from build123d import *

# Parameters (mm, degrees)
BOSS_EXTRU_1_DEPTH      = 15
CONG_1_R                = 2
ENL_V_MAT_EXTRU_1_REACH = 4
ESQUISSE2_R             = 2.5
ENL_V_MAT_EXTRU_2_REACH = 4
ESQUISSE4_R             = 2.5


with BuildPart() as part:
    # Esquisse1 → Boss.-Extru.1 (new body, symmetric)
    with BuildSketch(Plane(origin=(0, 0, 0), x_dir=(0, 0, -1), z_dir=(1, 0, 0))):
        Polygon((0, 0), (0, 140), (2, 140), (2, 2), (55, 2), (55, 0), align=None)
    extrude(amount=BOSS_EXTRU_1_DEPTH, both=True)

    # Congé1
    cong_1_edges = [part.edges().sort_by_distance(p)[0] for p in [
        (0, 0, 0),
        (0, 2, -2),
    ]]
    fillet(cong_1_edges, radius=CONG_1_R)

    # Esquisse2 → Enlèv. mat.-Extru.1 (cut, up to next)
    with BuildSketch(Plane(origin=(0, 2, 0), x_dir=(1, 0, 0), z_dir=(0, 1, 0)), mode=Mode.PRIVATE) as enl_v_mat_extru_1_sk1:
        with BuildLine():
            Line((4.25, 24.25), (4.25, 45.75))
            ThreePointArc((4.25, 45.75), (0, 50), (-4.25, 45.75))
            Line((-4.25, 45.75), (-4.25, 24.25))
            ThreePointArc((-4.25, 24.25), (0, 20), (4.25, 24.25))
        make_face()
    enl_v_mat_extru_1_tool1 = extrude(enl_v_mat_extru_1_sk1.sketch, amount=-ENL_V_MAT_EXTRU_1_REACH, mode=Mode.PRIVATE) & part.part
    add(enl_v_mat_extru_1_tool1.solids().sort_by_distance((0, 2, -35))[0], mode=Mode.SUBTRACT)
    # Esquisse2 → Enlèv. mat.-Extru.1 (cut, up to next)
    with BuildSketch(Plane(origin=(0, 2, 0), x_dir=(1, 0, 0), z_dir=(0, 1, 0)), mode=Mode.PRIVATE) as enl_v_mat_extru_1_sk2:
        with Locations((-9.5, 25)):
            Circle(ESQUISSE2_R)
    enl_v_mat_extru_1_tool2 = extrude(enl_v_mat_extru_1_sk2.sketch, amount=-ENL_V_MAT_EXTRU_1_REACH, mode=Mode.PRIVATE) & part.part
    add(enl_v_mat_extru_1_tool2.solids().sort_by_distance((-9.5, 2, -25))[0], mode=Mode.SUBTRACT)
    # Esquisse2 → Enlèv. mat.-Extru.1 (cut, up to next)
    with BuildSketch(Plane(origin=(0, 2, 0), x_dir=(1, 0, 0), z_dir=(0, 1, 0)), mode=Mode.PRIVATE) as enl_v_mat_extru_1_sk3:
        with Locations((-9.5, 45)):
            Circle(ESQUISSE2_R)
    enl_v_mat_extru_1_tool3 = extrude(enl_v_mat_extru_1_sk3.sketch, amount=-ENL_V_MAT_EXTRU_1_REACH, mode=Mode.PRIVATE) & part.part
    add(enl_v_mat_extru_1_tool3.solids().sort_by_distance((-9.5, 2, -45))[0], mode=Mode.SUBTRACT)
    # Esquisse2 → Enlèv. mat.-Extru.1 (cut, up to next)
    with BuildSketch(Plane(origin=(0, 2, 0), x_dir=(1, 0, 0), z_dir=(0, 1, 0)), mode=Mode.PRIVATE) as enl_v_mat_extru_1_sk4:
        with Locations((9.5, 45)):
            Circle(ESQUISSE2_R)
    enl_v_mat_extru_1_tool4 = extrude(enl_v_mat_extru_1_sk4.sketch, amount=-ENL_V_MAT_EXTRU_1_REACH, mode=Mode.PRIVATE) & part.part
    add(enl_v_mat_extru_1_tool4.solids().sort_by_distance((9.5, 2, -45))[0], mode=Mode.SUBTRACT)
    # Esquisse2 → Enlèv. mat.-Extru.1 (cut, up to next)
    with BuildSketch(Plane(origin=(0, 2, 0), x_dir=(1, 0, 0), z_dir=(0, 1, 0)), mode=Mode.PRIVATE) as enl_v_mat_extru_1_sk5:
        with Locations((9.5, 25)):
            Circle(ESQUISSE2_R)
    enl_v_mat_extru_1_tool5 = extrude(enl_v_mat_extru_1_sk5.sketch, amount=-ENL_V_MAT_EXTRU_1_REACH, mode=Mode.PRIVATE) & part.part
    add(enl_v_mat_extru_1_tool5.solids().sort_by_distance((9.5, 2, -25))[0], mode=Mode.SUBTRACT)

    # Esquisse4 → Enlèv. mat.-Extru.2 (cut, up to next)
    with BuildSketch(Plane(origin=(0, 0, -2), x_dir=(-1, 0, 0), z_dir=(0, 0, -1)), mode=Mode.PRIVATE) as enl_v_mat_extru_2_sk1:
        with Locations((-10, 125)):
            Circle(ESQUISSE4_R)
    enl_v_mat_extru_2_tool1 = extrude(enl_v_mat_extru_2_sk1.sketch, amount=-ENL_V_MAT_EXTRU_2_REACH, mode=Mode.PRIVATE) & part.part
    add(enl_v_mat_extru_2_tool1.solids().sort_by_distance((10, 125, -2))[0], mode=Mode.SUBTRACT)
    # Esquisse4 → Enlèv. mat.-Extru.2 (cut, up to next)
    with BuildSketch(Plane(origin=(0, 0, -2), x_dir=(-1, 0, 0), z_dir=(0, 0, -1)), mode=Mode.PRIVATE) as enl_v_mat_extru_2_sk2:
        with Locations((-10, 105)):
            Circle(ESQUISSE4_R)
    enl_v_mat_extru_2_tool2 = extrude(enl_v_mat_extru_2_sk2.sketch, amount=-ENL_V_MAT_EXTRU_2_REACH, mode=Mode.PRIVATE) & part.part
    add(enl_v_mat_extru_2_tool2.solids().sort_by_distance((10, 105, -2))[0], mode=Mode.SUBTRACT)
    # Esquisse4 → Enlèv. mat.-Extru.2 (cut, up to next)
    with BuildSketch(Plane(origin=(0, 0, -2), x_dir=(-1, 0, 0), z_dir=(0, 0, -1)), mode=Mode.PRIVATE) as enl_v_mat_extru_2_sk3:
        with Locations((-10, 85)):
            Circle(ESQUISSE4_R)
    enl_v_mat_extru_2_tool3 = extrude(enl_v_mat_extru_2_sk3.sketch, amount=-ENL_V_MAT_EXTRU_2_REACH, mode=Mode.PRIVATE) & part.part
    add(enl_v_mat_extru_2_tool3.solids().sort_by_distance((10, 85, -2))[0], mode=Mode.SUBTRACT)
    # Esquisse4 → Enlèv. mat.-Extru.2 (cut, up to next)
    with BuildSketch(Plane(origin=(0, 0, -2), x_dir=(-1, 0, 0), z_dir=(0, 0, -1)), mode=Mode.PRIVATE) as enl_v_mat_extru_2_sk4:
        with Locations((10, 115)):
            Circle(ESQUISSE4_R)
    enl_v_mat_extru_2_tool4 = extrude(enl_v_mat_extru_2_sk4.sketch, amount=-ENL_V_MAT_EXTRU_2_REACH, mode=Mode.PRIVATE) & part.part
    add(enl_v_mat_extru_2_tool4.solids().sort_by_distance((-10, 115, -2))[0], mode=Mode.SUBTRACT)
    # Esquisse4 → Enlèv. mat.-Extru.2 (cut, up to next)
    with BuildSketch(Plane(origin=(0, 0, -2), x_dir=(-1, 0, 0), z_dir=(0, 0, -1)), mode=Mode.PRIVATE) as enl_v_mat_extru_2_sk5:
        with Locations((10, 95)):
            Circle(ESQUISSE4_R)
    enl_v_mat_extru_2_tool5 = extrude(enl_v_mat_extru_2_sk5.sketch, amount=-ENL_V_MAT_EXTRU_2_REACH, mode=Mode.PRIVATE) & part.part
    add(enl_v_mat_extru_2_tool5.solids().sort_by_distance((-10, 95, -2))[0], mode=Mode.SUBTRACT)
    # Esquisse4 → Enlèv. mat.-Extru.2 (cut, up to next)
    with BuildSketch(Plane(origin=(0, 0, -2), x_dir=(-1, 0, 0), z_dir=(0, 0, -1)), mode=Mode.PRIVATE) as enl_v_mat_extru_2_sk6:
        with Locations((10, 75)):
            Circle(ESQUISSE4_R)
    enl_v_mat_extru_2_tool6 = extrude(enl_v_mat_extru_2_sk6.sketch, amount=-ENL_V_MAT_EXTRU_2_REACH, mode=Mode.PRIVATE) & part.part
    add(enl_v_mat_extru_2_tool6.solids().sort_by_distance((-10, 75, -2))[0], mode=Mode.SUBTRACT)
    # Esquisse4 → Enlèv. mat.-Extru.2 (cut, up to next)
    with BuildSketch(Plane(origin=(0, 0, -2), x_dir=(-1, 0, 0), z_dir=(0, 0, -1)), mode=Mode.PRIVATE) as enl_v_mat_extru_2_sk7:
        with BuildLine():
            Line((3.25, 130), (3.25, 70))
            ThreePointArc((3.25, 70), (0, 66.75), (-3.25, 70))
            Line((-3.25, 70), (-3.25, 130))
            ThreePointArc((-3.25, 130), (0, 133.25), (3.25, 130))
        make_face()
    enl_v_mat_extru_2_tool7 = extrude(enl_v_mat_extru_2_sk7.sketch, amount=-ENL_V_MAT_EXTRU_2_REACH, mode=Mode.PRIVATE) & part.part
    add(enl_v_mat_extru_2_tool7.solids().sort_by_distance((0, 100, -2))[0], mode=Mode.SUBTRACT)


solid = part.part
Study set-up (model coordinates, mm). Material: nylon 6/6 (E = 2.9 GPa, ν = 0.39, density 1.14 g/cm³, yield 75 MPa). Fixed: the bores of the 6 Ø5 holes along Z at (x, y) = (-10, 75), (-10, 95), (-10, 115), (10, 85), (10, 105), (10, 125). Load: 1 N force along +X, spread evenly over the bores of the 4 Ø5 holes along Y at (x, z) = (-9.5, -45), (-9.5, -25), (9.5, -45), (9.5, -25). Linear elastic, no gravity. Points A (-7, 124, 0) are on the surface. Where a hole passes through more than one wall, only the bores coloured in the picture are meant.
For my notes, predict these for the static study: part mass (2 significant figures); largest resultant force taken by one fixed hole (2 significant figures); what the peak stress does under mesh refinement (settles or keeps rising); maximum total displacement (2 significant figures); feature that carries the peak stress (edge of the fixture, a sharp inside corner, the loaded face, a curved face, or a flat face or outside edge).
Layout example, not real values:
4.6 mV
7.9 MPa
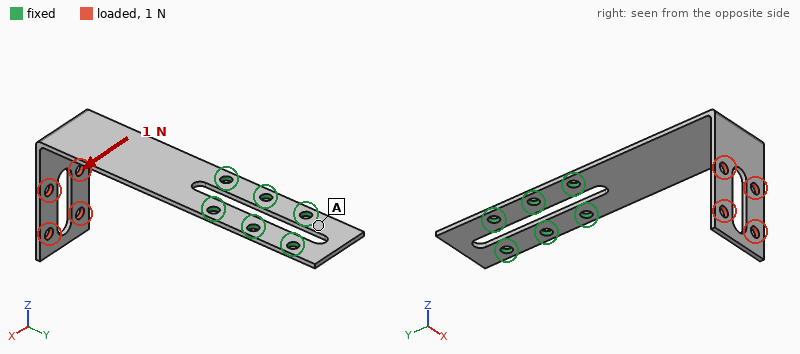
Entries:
11 g
3.5 N
keeps rising
1.7 mm
edge of the fixture
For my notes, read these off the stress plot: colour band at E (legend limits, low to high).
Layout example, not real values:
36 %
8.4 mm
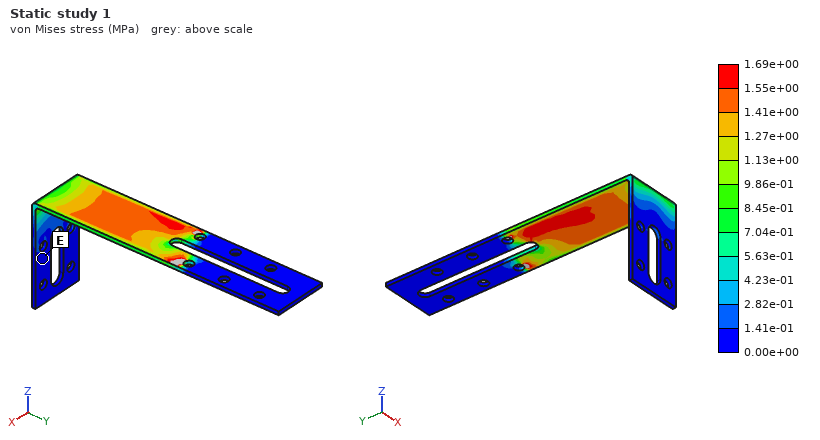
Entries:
0.00e+00 to 1.41e-01 MPa
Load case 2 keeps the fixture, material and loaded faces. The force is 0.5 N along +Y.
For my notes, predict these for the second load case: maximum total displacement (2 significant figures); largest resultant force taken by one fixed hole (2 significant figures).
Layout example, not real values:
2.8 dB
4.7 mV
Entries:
1.6 mm
0.37 N
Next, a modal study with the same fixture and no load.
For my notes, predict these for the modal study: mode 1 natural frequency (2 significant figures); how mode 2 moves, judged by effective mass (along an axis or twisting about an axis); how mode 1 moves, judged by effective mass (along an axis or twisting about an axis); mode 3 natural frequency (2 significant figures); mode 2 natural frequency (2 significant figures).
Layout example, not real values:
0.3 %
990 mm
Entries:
43 Hz
along X
along Z
140 Hz
99 Hz
